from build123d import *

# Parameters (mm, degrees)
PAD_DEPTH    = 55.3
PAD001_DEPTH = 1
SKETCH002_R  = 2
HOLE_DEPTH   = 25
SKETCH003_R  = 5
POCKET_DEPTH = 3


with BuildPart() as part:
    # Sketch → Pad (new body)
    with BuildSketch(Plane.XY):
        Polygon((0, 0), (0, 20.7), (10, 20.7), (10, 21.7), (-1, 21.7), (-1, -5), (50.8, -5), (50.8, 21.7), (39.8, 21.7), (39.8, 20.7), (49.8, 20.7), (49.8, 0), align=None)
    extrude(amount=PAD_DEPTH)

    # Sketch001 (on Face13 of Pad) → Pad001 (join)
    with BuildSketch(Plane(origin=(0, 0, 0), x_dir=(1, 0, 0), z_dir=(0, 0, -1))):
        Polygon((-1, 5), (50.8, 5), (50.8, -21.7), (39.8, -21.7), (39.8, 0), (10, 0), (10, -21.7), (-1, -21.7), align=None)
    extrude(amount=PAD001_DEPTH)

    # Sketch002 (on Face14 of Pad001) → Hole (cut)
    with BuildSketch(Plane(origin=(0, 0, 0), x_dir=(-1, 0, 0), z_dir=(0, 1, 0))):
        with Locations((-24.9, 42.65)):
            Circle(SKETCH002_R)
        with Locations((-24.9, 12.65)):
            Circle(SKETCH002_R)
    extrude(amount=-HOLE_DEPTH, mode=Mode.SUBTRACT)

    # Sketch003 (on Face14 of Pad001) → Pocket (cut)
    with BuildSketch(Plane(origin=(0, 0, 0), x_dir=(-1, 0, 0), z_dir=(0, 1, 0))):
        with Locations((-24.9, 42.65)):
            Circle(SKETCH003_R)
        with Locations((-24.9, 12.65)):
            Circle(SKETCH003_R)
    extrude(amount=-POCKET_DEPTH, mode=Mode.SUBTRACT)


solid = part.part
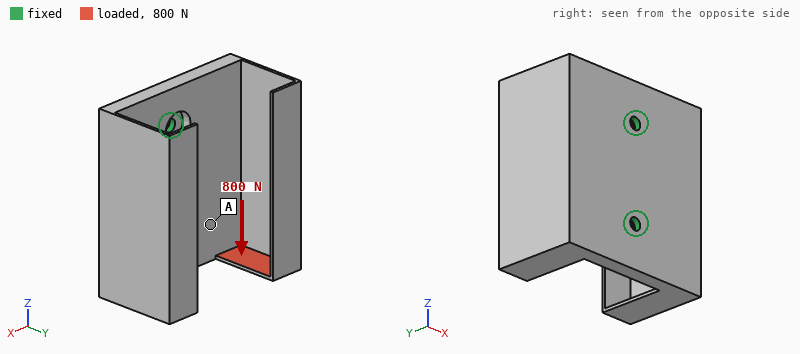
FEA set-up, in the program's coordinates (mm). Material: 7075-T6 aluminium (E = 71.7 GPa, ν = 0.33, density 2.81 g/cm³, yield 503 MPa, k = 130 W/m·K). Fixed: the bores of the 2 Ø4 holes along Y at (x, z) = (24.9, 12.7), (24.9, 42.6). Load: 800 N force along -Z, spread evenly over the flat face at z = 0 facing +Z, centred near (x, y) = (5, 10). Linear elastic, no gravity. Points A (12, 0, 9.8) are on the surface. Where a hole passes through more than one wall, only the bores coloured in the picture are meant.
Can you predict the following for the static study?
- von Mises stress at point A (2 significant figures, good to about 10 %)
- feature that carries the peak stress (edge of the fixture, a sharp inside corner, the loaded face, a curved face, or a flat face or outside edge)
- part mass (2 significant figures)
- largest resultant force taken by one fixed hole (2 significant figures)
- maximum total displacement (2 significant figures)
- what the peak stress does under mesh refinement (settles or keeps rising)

37 MPa
a sharp inside corner
51 g
750 N
0.80 mm
keeps rising
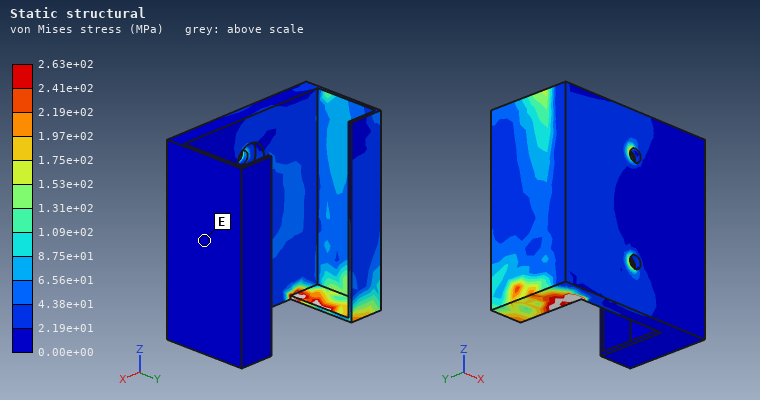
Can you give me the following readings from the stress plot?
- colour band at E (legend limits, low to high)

0.00e+00 to 2.19e+01 MPa
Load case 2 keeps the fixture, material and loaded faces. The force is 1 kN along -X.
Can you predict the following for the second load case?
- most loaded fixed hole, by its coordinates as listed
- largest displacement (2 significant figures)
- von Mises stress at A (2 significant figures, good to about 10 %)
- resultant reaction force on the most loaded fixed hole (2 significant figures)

(24.9, 12.7)
0.92 mm
99 MPa
1.4 kN
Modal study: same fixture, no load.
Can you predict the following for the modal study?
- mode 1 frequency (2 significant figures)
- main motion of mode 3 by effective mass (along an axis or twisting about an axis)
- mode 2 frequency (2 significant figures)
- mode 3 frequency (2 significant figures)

1200 Hz
twisting about Z
1300 Hz
1700 Hz
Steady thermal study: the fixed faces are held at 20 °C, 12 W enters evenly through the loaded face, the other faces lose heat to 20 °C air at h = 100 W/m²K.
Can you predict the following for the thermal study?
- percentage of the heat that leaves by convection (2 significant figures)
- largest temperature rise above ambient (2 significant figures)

55 %
40 K
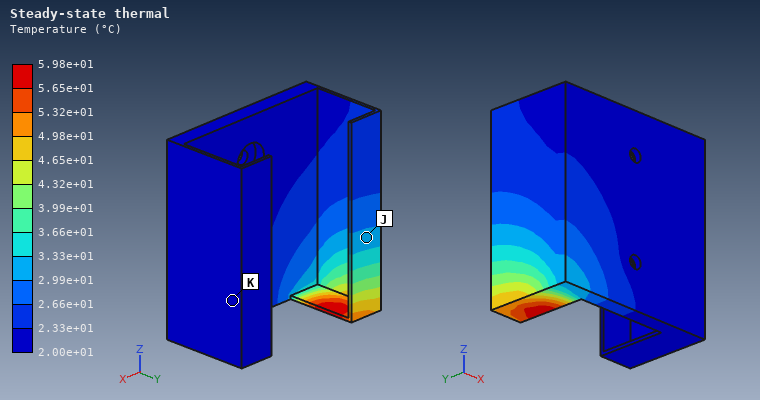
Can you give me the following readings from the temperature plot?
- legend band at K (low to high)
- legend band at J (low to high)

2.00e+01 to 2.33e+01 °C
2.99e+01 to 3.33e+01 °C
